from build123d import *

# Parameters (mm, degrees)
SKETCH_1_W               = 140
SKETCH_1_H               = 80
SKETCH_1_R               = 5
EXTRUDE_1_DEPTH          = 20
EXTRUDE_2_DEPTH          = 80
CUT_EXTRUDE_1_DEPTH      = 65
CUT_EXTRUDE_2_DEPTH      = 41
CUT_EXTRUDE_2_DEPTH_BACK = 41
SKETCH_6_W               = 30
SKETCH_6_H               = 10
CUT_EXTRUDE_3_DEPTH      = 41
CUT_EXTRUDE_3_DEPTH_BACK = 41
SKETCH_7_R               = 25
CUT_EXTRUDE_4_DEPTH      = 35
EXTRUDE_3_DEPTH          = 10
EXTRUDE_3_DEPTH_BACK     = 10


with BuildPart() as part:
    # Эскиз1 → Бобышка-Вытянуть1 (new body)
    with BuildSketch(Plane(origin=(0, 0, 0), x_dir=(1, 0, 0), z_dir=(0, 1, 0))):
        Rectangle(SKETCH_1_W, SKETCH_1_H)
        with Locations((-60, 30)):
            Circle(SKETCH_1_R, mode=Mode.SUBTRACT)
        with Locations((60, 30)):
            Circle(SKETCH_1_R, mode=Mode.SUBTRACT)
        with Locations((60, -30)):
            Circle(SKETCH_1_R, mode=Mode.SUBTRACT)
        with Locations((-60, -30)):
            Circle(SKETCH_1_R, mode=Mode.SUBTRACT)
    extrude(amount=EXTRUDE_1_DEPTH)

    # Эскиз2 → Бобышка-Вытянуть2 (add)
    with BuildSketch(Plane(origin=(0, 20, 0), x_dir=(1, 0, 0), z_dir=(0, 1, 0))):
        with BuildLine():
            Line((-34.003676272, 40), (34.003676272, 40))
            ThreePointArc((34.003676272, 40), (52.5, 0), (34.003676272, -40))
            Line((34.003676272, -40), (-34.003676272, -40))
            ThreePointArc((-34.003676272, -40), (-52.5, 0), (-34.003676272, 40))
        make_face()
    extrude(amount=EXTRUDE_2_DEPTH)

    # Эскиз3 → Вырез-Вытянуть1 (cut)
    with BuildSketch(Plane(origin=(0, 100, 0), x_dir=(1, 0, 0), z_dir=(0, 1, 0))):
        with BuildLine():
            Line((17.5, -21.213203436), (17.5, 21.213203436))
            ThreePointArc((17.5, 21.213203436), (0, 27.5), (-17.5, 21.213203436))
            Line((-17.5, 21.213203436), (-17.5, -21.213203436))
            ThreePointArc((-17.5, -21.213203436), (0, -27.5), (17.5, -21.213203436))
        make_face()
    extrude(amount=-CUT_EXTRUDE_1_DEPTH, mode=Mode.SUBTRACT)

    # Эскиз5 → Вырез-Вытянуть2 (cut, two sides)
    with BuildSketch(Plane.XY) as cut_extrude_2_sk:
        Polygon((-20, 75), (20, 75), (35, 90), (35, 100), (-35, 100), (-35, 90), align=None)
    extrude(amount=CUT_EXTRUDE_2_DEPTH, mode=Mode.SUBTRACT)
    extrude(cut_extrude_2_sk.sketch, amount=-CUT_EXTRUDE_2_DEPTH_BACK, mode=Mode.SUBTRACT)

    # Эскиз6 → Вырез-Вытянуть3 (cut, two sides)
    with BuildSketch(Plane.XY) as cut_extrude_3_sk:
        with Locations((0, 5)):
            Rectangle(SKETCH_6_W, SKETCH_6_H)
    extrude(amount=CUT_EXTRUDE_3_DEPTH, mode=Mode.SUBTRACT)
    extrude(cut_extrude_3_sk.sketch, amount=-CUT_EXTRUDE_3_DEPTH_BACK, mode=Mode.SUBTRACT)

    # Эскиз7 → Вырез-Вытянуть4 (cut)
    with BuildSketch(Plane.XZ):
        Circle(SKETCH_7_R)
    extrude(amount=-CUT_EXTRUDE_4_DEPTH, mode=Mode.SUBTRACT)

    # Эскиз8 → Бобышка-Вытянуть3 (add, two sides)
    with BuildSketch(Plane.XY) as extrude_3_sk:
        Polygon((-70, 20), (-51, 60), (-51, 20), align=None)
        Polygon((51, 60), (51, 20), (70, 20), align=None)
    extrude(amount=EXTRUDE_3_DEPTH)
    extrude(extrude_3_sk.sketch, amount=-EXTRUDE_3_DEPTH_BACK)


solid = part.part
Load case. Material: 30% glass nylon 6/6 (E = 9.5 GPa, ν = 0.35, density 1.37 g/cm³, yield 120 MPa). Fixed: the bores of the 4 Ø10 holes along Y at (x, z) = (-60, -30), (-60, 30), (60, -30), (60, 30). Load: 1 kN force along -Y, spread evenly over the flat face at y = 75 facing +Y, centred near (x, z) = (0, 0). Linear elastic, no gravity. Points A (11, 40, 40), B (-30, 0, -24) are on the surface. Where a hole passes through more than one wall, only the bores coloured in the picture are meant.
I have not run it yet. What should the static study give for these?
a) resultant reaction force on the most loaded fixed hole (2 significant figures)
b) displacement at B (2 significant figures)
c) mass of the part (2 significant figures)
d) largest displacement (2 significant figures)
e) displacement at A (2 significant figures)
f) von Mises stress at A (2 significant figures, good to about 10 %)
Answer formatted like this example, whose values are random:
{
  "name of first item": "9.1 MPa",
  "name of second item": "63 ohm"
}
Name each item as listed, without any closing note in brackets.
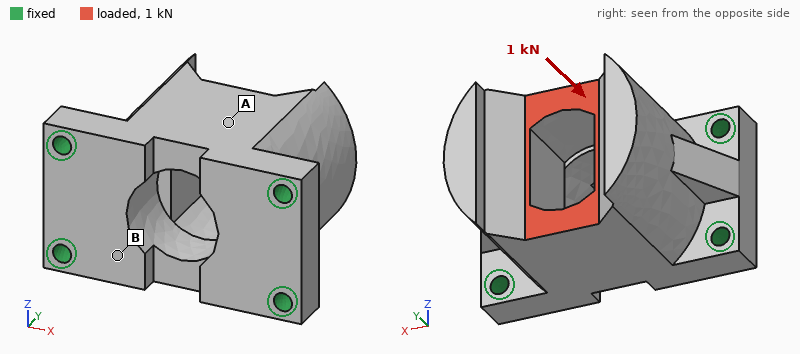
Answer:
{
  "resultant reaction force on the most loaded fixed hole": "310 N",
  "displacement at B": "4.3 µm",
  "mass of the part": "770 g",
  "largest displacement": "8.4 µm",
  "displacement at A": "5.9 µm",
  "von Mises stress at A": "0.41 MPa"
}
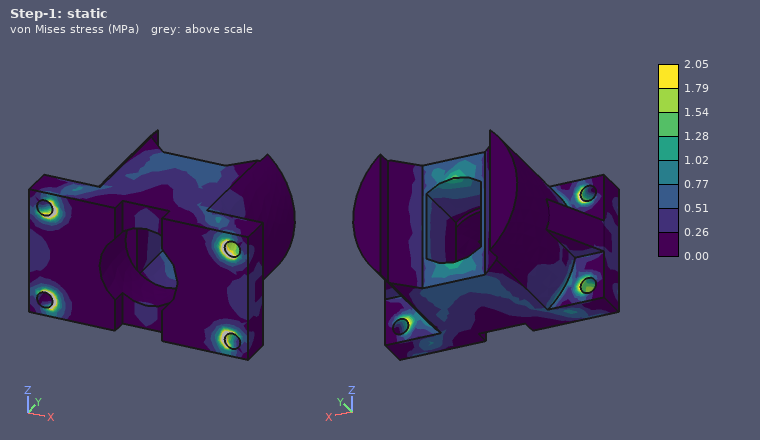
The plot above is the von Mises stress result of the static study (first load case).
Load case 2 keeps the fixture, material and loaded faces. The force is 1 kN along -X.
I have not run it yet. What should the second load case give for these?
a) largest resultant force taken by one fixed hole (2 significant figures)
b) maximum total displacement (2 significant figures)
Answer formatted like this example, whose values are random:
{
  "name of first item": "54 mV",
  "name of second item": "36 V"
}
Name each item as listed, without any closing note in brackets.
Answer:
{
  "largest resultant force taken by one fixed hole": "390 N",
  "maximum total displacement": "13 µm"
}
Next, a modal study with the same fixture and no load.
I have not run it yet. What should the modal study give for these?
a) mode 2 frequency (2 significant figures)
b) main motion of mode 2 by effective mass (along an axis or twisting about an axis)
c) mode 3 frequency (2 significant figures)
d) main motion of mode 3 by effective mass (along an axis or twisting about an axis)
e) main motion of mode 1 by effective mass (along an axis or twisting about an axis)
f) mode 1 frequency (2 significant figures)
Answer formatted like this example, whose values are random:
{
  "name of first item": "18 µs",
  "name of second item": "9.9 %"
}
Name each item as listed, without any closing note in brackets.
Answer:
{
  "mode 2 frequency": "2700 Hz",
  "main motion of mode 2 by effective mass": "along X",
  "mode 3 frequency": "3000 Hz",
  "main motion of mode 3 by effective mass": "along Y",
  "main motion of mode 1 by effective mass": "along Z",
  "mode 1 frequency": "1700 Hz"
}
